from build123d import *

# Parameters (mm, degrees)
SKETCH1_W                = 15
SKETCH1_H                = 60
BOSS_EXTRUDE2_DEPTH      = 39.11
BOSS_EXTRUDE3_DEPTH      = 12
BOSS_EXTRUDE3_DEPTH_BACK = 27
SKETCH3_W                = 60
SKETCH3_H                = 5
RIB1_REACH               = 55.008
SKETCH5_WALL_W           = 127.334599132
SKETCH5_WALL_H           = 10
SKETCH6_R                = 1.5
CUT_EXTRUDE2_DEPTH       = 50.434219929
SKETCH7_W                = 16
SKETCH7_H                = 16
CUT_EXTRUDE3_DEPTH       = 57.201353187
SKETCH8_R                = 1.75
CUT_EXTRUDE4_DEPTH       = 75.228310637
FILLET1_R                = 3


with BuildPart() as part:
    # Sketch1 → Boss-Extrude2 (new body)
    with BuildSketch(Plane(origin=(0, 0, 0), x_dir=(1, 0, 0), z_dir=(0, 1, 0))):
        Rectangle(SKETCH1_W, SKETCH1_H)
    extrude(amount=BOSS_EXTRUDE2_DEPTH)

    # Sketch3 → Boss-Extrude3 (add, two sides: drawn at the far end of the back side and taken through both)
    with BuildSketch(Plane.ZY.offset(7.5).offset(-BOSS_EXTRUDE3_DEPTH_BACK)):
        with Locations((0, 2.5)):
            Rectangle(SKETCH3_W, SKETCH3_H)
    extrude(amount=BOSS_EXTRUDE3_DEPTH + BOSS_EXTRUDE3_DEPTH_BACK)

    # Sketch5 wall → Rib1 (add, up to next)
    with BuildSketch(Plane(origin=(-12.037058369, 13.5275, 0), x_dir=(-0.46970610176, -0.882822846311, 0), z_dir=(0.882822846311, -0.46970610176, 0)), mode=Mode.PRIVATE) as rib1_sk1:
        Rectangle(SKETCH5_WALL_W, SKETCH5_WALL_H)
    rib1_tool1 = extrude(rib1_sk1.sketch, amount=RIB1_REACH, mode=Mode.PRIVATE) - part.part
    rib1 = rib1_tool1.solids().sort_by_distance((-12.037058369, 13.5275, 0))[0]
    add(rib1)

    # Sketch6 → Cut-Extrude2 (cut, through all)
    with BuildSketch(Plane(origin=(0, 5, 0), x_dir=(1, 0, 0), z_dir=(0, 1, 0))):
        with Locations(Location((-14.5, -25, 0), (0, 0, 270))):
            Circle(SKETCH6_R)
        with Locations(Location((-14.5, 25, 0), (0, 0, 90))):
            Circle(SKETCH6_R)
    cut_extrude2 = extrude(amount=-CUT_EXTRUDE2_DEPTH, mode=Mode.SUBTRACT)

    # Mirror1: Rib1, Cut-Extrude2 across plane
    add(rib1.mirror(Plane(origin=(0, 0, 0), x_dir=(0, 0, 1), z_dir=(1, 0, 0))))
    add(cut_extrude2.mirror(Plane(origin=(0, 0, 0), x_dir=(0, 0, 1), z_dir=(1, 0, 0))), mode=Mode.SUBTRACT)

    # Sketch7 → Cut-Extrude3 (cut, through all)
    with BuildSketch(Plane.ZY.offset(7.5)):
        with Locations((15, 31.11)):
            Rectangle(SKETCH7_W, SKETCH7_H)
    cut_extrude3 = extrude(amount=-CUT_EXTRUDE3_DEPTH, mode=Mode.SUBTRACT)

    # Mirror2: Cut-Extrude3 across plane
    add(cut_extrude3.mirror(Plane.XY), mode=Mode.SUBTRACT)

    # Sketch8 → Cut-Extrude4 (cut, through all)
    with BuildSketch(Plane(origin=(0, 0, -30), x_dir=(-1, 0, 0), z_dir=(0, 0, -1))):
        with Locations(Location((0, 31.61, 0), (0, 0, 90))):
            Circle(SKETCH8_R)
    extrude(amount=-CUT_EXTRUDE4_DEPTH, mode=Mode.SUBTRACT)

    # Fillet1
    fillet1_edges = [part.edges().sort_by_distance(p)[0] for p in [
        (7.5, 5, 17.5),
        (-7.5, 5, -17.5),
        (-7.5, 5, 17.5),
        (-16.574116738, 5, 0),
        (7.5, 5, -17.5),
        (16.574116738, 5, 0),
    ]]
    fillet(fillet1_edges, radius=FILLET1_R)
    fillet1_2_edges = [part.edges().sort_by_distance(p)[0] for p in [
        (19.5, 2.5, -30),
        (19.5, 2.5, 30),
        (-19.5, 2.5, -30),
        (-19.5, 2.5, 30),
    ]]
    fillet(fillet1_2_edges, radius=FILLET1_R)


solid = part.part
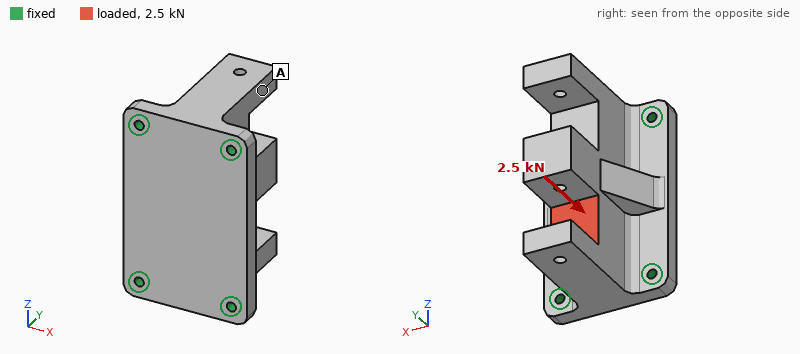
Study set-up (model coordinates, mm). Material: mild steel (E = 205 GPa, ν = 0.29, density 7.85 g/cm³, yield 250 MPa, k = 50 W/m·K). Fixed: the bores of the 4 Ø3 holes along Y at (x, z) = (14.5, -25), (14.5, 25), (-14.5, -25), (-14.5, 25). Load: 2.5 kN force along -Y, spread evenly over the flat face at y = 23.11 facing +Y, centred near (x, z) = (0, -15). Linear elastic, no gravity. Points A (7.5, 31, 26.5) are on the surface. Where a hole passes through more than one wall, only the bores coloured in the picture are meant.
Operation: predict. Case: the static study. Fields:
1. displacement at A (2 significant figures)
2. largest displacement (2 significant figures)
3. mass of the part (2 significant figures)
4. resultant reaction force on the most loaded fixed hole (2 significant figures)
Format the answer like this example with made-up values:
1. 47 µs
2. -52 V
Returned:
1. 2.2 µm
2. 4.4 µm
3. 280 g
4. 1.1 kN
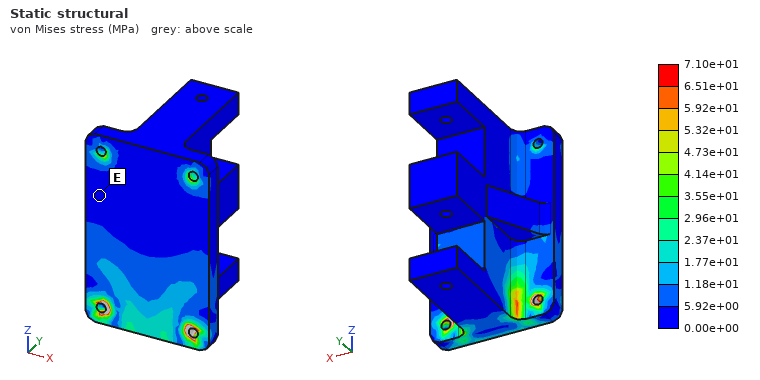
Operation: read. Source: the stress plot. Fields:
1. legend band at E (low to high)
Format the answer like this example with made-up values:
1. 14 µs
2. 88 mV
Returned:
1. 0.00e+00 to 5.92e+00 MPa
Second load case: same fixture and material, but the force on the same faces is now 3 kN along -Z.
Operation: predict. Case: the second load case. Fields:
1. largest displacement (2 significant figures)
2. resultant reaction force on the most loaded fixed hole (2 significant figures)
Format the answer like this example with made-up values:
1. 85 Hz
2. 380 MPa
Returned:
1. 8.6 µm
2. 1.1 kN
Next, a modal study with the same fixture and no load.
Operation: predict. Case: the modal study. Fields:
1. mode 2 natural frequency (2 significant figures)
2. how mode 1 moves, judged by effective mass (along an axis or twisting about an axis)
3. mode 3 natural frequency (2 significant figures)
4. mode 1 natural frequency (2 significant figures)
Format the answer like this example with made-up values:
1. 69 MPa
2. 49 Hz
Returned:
1. 9300 Hz
2. along X
3. 9400 Hz
4. 6400 Hz
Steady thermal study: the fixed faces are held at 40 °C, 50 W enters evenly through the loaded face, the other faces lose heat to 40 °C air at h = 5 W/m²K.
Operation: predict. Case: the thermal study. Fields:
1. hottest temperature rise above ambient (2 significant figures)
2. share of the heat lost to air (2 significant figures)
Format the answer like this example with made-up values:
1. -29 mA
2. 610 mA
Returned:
1. 79 K
2. 3.5 %
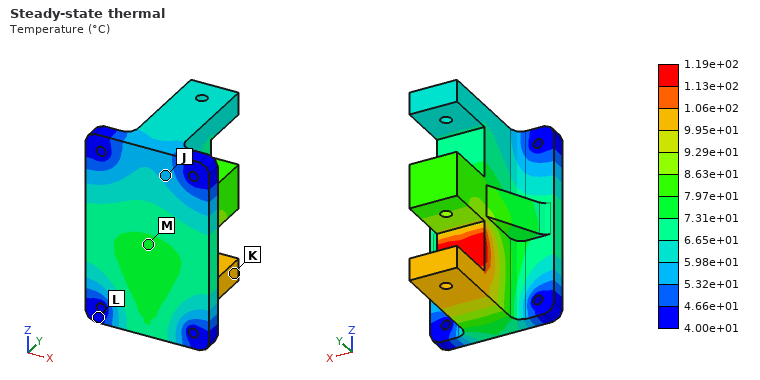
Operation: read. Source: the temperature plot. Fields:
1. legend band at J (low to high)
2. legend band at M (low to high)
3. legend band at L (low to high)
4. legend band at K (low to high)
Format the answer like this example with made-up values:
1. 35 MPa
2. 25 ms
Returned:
1. 5.32e+01 to 5.98e+01 °C
2. 7.31e+01 to 7.97e+01 °C
3. 4.00e+01 to 4.66e+01 °C
4. 9.95e+01 to 1.06e+02 °C
